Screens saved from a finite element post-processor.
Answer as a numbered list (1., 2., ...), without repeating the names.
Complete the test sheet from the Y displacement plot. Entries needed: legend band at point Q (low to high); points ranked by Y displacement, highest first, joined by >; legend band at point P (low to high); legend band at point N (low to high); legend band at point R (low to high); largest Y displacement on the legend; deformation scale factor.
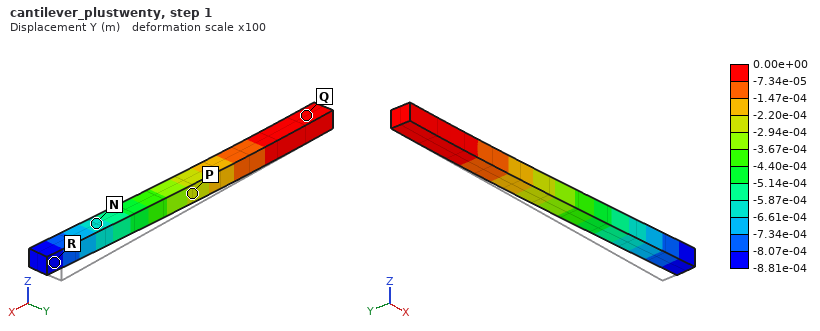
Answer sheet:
1. -7.34e-05 to 0.00e+00 m
2. Q > P > N > R
3. -2.94e-04 to -2.20e-04 m
4. -6.61e-04 to -5.87e-04 m
5. -8.81e-04 to -8.07e-04 m
6. 0.00e+00 m
7. 100
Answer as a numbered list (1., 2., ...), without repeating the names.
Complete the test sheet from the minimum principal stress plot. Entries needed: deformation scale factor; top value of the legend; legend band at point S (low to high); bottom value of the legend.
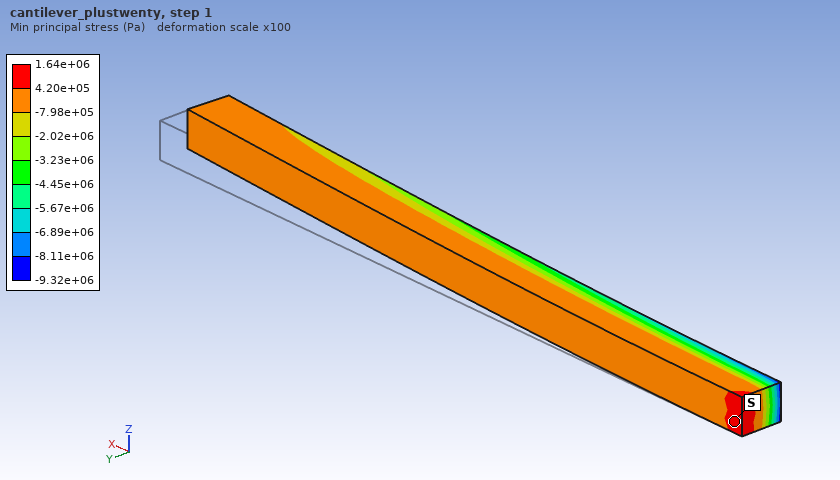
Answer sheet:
1. 100
2. 1.64e+06 Pa
3. 4.20e+05 to 1.64e+06 Pa
4. -9.32e+06 Pa
